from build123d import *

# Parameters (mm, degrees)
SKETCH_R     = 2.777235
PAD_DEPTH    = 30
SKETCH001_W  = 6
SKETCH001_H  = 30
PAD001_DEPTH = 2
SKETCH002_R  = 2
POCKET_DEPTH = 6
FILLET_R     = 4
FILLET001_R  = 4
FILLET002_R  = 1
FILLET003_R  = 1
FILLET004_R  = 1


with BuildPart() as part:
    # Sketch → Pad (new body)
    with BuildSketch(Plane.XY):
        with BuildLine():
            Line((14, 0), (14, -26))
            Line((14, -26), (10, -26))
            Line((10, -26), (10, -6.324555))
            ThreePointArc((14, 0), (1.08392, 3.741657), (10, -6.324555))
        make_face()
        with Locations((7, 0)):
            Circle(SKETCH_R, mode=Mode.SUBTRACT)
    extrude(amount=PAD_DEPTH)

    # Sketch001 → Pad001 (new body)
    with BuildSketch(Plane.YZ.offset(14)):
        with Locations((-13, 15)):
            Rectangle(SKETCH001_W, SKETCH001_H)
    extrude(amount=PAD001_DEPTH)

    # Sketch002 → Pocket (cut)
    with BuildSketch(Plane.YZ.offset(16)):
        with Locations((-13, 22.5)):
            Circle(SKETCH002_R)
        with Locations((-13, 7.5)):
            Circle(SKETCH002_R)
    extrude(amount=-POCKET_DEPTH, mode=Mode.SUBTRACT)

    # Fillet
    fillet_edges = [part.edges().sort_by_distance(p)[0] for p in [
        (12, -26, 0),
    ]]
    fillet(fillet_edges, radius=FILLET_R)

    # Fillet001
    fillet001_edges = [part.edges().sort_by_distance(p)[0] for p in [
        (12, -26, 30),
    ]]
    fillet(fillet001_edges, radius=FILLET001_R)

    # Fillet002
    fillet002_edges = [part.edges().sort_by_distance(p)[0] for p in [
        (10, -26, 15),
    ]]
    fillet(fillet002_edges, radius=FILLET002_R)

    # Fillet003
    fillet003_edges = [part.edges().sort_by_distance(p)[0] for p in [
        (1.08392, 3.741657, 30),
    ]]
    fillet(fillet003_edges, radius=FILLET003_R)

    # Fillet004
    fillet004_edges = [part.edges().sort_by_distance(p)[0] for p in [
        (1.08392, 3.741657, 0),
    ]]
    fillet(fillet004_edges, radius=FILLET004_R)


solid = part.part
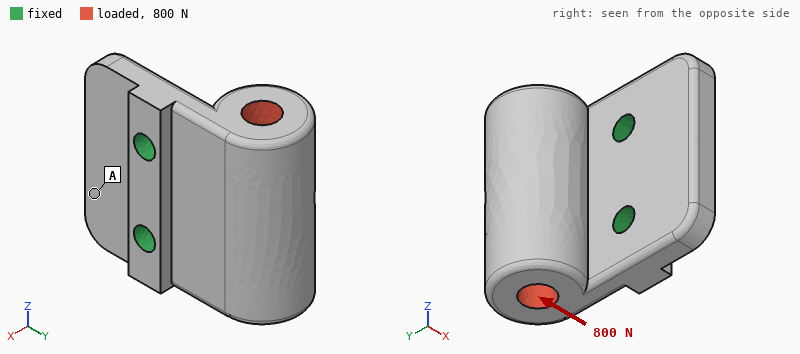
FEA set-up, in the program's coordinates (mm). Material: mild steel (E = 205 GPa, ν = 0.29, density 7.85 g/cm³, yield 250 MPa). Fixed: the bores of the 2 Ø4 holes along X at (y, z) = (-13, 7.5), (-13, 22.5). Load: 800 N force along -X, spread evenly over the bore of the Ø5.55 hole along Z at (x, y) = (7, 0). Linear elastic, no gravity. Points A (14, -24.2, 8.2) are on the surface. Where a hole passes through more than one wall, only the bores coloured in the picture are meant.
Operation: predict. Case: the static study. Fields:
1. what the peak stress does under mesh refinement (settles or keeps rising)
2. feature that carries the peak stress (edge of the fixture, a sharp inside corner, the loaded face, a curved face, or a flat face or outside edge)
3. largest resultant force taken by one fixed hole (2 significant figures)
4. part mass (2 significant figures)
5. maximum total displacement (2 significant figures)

keeps rising
edge of the fixture
400 N
52 g
25 µm
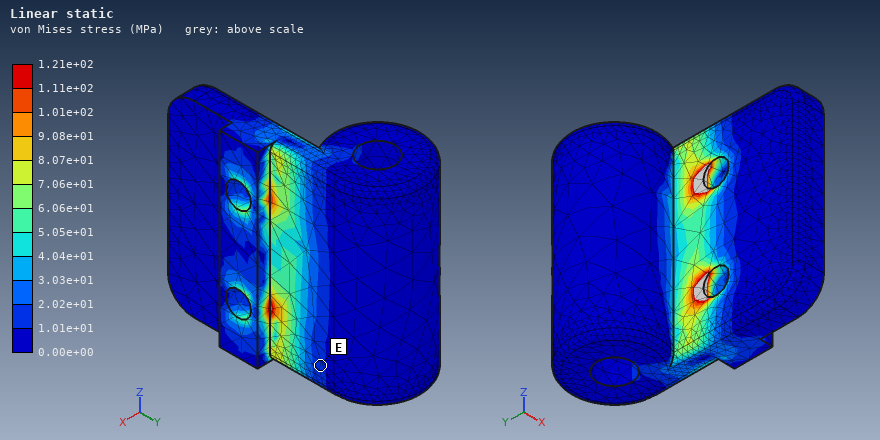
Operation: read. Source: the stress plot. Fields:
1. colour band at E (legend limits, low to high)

1.01e+01 to 2.02e+01 MPa
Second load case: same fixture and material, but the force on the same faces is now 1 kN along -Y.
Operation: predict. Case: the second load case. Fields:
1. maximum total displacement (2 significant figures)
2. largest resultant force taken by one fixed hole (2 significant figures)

19 µm
500 N
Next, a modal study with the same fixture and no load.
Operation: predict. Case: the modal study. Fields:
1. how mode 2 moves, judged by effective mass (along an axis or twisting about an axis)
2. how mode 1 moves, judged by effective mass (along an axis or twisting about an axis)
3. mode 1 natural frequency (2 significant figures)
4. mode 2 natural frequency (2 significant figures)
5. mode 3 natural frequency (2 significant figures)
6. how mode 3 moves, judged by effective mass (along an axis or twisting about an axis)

along Z
along X
5400 Hz
14 kHz
20 kHz
along Z
